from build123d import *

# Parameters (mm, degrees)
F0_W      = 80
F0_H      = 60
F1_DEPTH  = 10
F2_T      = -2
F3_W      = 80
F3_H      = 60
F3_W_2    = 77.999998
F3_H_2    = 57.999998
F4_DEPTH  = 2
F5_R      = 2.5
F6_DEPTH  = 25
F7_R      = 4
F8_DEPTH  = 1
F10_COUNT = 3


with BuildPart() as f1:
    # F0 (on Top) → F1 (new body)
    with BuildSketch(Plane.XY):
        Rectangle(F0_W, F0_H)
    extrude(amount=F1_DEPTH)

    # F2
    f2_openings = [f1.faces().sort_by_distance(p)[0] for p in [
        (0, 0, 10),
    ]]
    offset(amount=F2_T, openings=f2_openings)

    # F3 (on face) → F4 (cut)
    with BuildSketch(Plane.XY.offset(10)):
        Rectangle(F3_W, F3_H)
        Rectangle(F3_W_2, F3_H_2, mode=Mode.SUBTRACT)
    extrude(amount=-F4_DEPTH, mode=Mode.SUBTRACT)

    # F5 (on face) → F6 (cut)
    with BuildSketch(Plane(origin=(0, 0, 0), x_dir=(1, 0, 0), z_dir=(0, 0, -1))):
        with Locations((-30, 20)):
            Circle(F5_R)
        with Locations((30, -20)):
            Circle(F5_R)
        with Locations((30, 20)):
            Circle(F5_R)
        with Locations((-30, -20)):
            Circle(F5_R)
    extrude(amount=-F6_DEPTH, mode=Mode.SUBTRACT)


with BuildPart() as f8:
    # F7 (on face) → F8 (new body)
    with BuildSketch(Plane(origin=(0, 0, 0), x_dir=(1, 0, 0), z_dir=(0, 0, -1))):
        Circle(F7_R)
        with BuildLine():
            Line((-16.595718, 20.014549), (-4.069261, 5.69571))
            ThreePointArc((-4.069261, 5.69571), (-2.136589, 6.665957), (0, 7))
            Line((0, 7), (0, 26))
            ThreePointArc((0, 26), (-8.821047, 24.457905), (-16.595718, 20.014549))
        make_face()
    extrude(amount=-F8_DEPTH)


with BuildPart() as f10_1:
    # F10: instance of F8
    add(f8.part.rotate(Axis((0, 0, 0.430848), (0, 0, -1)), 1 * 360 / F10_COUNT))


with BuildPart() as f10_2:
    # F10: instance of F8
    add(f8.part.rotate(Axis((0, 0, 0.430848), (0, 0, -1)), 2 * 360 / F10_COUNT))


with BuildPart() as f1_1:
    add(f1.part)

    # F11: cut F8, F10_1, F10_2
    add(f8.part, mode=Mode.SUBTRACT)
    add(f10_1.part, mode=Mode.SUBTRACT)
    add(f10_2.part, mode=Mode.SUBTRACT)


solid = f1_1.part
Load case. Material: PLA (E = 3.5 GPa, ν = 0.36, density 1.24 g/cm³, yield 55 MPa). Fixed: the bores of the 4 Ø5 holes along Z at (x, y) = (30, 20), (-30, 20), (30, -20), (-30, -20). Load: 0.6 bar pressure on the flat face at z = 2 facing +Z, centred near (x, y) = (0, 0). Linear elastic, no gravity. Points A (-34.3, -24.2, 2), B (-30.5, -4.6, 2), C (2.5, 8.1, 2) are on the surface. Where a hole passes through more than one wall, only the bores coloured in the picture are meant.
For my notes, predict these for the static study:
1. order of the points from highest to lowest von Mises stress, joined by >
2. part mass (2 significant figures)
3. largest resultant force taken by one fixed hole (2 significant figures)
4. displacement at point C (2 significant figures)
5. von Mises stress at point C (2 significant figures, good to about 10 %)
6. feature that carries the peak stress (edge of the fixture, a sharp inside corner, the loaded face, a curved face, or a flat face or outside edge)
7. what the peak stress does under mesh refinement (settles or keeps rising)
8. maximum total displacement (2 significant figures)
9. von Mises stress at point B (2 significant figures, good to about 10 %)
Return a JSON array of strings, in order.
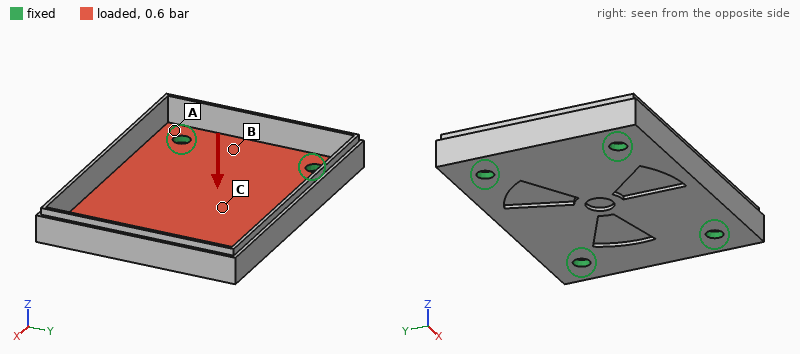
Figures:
["C > B > A", "16 g", "82 N", "0.82 mm", "8.8 MPa", "edge of the fixture", "keeps rising", "0.97 mm", "6.3 MPa"]
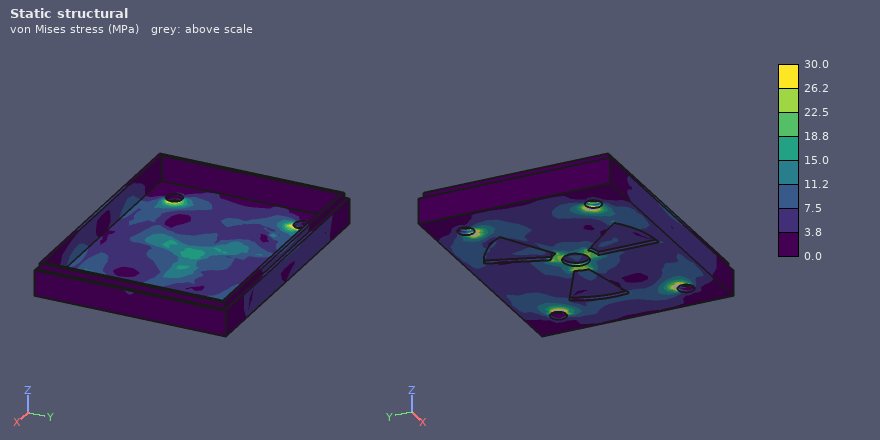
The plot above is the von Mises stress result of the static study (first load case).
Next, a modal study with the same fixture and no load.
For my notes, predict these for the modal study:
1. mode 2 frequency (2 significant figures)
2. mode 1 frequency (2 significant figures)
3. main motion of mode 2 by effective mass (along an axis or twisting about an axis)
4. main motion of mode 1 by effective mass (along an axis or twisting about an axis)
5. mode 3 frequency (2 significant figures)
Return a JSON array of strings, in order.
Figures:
["1900 Hz", "1100 Hz", "twisting about X", "along Z", "2000 Hz"]
